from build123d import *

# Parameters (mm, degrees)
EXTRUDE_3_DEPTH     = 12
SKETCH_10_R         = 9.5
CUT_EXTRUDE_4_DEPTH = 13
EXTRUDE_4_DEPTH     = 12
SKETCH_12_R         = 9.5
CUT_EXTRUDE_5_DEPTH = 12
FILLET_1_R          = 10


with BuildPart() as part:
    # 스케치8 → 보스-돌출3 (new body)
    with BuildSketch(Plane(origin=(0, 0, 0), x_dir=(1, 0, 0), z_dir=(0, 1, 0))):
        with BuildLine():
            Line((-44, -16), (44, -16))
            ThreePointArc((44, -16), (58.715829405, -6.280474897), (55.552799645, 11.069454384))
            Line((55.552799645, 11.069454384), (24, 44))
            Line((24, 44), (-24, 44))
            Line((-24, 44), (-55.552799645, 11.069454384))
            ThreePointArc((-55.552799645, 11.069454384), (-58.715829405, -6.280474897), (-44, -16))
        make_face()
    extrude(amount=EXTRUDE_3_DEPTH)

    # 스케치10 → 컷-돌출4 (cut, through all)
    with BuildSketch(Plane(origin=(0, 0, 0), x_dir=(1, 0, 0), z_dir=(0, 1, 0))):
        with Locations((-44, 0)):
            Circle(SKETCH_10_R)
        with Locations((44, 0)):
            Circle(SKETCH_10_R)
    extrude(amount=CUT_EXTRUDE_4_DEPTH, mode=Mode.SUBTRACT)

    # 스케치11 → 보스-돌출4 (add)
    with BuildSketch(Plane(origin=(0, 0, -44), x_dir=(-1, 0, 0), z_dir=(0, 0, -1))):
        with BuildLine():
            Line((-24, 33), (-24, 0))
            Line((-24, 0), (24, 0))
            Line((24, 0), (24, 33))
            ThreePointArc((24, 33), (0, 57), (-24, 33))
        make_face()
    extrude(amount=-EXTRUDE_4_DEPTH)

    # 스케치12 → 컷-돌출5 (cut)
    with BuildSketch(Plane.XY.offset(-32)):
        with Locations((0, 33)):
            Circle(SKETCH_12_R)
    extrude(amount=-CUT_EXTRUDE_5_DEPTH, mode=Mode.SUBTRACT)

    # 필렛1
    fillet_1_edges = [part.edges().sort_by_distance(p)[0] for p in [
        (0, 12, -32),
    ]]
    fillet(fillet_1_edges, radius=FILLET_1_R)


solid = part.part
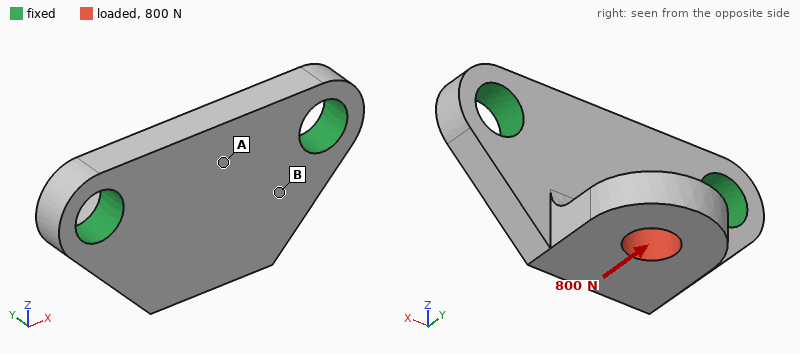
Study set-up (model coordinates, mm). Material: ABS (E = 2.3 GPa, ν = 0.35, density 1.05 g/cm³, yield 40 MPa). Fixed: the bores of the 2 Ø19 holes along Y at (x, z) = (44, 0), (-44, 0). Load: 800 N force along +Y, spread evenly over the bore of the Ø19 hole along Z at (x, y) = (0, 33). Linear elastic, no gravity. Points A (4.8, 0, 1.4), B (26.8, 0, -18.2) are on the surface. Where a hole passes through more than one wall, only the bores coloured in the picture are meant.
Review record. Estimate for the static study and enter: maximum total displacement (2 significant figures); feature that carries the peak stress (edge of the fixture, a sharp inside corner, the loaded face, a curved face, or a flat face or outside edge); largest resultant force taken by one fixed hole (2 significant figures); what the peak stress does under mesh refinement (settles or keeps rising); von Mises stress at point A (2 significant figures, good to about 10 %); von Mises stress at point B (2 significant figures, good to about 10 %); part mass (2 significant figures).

1.3 mm
edge of the fixture
400 N
keeps rising
2.5 MPa
8.0 MPa
87 g
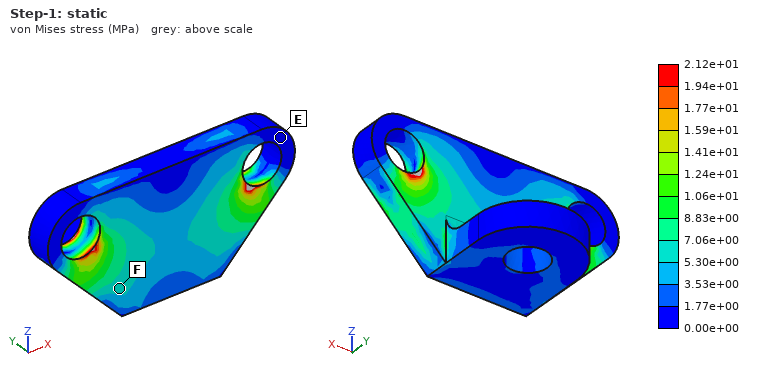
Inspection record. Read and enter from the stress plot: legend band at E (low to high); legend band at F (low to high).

0.00e+00 to 1.77e+00 MPa
5.30e+00 to 7.06e+00 MPa
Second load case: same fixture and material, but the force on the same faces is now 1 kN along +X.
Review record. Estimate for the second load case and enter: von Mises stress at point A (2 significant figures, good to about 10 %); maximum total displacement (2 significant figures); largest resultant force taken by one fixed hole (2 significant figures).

1.5 MPa
0.61 mm
750 N
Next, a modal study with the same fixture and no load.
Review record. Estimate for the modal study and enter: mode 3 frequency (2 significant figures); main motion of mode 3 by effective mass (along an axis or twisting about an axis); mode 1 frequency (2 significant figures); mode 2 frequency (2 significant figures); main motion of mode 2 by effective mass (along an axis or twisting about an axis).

1600 Hz
along Y
730 Hz
1500 Hz
along X
